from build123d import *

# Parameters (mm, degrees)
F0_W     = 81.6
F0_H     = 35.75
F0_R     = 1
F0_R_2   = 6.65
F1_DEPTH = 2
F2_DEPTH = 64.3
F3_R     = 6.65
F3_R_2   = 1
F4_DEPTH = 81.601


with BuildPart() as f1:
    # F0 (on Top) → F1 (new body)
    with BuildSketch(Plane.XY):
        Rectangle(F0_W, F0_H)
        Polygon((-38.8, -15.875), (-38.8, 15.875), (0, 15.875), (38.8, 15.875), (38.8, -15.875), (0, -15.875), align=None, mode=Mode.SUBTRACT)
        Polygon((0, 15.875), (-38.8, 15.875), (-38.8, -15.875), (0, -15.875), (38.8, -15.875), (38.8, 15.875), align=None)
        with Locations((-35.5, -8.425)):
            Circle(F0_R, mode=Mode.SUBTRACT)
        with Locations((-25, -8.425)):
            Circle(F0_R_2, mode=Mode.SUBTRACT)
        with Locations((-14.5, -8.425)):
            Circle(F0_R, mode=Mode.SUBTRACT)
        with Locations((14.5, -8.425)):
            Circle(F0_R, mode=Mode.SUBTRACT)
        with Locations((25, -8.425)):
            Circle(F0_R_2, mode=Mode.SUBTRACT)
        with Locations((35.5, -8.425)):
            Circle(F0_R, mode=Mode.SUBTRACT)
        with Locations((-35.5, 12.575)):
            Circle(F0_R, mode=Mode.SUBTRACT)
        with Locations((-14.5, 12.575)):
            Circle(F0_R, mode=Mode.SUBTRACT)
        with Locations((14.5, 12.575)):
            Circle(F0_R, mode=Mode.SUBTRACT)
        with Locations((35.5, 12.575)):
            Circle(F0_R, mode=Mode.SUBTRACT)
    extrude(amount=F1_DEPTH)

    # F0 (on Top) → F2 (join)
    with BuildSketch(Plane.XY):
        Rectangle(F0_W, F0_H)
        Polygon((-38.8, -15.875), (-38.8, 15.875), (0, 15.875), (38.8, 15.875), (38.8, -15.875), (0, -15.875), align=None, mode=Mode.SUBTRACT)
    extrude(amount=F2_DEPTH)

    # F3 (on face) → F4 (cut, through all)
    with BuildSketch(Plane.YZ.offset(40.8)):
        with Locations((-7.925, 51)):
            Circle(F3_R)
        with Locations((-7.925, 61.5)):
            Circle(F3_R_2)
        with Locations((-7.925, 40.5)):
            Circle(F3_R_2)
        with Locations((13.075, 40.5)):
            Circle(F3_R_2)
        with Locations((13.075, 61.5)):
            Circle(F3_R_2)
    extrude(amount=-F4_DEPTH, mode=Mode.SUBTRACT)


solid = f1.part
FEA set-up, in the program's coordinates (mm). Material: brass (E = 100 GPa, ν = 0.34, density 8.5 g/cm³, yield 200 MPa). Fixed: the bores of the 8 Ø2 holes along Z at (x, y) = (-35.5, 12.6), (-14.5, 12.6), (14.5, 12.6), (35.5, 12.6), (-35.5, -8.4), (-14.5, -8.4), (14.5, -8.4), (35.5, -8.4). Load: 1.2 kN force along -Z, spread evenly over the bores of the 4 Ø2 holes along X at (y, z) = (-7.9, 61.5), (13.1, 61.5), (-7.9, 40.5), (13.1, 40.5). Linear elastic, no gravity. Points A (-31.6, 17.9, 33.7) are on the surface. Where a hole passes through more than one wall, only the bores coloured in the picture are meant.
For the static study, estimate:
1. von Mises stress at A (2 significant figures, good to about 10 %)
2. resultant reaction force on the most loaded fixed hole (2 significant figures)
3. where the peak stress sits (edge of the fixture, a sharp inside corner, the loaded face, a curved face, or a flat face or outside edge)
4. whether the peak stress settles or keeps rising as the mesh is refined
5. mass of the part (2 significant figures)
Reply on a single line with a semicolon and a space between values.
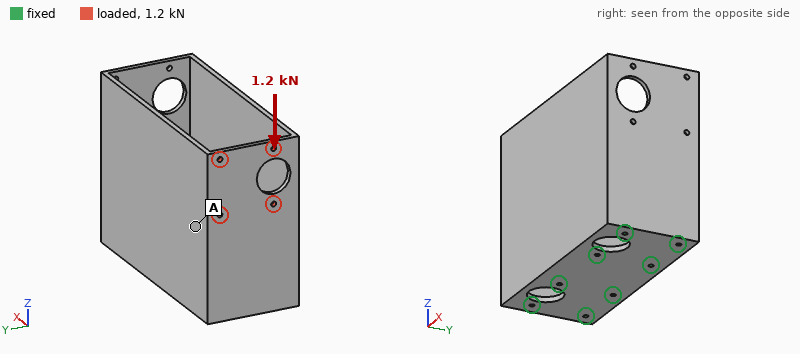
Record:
7.8 MPa; 550 N; edge of the fixture; keeps rising; 280 g
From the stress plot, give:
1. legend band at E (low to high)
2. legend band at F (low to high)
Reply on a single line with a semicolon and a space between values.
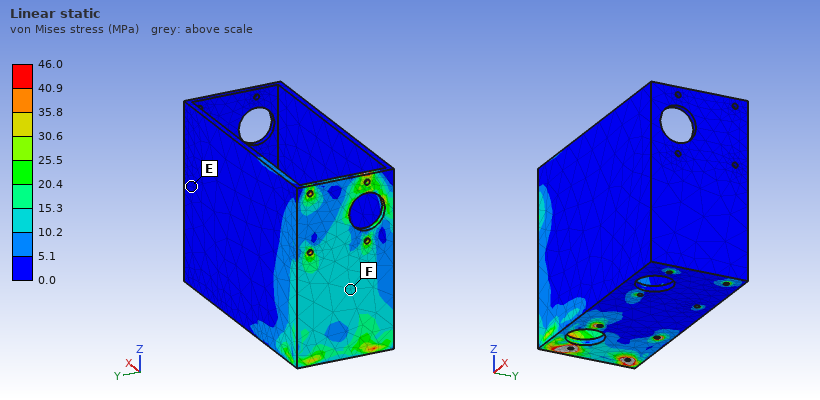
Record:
0.0 to 5.1 MPa; 10.2 to 15.3 MPa
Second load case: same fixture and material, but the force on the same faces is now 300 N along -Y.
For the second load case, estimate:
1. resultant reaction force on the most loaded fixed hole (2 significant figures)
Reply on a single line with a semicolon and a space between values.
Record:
550 N
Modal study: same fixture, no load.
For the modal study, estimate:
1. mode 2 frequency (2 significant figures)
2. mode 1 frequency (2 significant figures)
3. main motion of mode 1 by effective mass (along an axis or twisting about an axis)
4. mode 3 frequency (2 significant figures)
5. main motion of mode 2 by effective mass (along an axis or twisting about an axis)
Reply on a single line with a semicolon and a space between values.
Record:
950 Hz; 900 Hz; along Y; 1500 Hz; along Y
